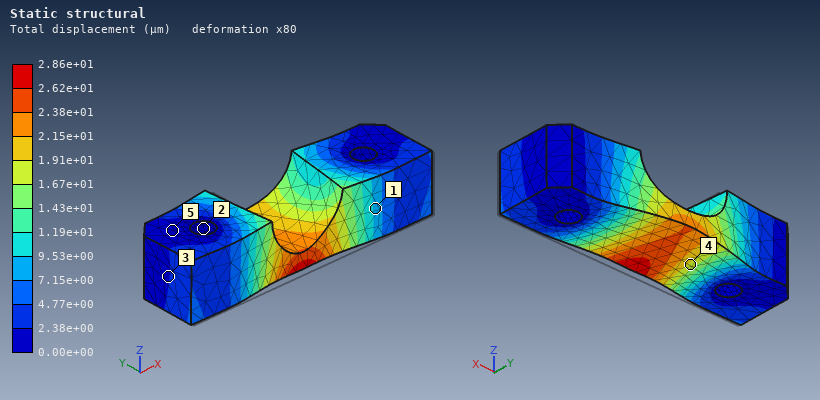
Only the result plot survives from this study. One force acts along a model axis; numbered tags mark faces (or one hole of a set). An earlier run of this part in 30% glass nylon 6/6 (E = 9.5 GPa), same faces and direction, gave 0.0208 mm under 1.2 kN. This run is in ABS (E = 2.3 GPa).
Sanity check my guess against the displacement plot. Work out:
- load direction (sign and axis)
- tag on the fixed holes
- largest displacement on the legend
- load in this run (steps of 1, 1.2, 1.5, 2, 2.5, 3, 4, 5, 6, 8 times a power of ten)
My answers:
+Y
2
2.86e+01 µm
400 N
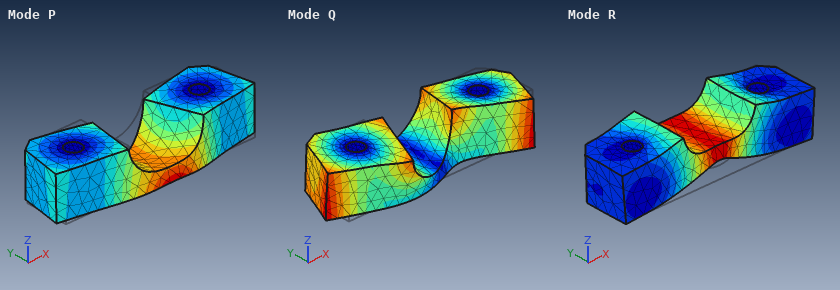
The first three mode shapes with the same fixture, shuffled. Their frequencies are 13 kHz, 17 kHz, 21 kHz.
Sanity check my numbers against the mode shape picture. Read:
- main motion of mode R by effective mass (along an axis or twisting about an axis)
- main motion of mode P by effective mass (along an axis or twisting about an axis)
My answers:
along Z
along Y
